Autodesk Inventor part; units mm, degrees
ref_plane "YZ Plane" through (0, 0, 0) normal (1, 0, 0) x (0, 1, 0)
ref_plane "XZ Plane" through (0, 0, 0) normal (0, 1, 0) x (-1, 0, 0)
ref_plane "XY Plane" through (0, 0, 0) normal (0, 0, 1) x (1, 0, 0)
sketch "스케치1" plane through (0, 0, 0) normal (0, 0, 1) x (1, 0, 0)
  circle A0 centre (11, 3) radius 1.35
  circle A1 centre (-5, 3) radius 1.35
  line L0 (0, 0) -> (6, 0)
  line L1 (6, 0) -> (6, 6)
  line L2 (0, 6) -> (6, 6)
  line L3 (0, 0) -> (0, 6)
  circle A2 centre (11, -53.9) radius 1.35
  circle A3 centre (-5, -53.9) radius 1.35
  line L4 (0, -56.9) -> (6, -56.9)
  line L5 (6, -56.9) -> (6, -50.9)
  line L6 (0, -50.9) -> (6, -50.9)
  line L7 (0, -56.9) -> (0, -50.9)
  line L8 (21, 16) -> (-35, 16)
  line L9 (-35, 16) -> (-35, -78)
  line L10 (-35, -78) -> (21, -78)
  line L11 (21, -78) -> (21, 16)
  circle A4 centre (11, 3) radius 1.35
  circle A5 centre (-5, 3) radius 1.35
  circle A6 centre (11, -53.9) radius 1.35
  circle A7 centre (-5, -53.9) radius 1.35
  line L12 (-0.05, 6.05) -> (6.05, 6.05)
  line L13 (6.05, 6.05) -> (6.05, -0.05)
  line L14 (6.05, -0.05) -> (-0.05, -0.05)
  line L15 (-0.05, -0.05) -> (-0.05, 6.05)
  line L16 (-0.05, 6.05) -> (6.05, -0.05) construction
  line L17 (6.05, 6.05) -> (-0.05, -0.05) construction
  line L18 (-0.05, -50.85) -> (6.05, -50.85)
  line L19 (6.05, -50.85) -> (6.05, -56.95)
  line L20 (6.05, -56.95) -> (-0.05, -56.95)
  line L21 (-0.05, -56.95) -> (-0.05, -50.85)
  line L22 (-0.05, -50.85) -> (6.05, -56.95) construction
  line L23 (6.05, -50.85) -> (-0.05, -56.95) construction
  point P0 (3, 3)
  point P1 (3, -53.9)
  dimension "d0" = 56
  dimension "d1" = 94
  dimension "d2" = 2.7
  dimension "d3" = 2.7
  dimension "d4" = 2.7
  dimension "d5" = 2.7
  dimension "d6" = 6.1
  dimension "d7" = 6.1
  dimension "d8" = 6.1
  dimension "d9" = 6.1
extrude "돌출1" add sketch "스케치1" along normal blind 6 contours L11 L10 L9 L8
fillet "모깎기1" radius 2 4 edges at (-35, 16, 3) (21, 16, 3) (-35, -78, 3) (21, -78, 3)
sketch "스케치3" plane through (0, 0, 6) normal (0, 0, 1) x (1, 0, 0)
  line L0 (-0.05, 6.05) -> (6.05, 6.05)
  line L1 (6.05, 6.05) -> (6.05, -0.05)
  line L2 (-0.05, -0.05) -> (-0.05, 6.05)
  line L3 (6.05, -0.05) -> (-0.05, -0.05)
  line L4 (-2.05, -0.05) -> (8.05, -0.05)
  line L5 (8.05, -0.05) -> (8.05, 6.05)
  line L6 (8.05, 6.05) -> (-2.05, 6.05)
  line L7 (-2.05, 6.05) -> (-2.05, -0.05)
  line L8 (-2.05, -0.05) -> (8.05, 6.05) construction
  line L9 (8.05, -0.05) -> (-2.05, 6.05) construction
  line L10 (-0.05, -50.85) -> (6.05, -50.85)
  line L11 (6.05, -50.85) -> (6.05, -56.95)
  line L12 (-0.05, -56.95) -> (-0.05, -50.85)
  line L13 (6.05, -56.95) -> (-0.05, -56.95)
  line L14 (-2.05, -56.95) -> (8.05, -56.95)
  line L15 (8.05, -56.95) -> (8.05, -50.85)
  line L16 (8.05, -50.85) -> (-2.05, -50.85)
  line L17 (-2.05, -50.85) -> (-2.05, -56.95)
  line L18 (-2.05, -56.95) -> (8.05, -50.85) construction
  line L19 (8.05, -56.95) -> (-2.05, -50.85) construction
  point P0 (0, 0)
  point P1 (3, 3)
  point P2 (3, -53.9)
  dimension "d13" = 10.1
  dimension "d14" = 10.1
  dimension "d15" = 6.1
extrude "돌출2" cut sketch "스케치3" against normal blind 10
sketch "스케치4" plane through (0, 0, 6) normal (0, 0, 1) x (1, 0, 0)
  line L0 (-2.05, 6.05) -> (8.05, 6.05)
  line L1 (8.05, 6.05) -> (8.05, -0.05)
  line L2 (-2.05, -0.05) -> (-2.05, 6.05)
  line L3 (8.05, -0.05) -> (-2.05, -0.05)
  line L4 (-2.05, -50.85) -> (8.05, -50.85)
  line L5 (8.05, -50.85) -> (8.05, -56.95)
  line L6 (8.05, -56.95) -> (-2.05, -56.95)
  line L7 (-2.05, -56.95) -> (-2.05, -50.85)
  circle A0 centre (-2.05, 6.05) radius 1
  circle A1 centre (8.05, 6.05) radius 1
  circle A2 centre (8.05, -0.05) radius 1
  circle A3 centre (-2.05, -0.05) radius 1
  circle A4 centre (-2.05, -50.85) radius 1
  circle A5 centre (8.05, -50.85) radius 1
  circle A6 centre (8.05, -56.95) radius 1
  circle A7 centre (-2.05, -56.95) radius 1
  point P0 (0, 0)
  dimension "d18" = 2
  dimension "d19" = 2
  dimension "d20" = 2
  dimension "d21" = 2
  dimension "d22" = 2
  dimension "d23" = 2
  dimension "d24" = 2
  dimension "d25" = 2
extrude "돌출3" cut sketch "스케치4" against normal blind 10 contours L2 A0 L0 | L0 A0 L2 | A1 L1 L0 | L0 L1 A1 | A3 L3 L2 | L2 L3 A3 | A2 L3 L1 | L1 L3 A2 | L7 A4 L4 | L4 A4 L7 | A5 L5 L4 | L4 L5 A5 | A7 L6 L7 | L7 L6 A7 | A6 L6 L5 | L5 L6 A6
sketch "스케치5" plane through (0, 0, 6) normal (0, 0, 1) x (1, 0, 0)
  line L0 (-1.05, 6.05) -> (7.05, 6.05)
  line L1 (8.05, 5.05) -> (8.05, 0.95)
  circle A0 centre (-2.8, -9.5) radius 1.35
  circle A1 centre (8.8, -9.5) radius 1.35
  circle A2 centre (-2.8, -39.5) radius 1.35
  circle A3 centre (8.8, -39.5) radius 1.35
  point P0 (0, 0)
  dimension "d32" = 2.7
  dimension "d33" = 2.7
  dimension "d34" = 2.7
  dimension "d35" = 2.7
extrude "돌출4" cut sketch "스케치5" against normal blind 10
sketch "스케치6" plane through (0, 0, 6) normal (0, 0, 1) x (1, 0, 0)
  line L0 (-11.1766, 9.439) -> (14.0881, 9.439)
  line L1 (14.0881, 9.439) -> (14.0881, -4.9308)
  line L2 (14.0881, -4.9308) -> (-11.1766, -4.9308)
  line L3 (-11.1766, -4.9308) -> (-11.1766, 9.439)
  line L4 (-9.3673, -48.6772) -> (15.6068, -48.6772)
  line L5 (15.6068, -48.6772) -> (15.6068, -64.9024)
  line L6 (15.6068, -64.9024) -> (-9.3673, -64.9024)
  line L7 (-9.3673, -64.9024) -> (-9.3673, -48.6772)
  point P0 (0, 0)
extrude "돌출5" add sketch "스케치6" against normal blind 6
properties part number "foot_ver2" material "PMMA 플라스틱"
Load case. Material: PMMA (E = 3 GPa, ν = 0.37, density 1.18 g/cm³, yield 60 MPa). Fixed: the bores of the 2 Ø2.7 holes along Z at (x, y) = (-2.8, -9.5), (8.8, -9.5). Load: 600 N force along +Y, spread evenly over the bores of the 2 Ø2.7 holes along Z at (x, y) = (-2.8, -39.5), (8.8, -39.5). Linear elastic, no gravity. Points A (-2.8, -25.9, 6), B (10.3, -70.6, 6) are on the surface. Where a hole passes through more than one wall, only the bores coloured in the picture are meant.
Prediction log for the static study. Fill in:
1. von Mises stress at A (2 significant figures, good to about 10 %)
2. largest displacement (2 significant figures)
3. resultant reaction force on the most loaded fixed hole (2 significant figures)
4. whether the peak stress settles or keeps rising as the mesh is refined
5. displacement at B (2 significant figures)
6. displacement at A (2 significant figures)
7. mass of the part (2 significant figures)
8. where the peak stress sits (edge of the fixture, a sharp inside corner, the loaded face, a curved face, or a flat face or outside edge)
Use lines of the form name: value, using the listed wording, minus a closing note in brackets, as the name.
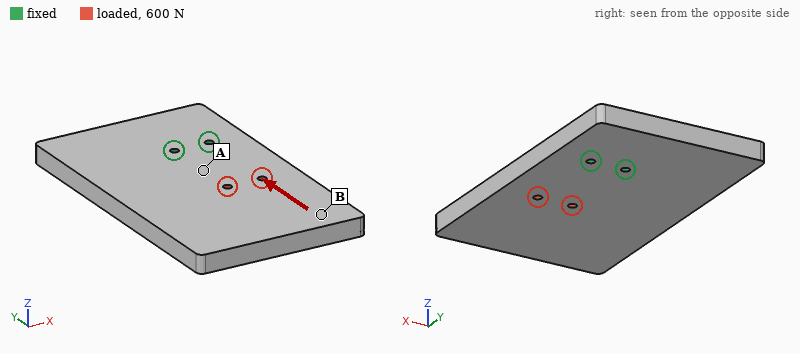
von Mises stress at A: 3.3 MPa
largest displacement: 42 µm
resultant reaction force on the most loaded fixed hole: 300 N
whether the peak stress settles or keeps rising as the mesh is refined: keeps rising
displacement at B: 37 µm
displacement at A: 20 µm
mass of the part: 37 g
where the peak stress sits: edge of the fixture
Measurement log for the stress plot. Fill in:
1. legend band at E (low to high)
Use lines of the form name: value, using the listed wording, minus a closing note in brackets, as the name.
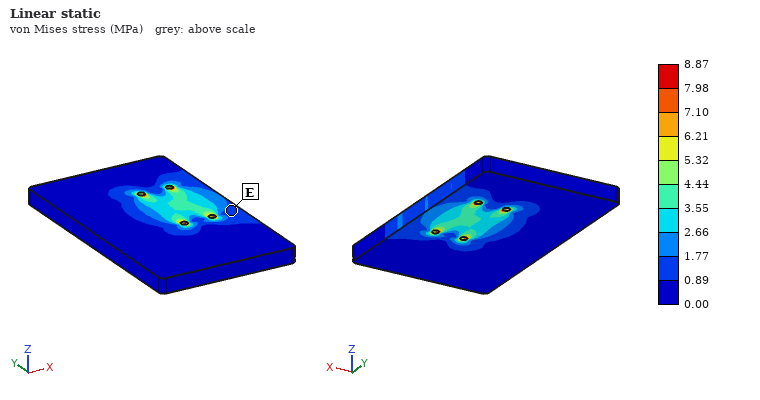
legend band at E: 0.89 to 1.77 MPa
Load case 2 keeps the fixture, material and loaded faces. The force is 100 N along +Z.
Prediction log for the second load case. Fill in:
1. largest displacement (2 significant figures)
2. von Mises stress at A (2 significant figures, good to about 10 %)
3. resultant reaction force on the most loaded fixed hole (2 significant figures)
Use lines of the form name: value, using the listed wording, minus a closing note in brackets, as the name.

largest displacement: 1.3 mm
von Mises stress at A: 4.2 MPa
resultant reaction force on the most loaded fixed hole: 50 N
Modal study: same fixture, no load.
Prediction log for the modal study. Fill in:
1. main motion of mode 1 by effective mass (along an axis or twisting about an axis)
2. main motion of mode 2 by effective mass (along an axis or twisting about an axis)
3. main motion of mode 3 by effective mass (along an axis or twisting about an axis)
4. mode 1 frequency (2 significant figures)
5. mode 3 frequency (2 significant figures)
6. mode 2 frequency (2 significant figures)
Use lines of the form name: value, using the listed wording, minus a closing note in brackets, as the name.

main motion of mode 1 by effective mass: along Z
main motion of mode 2 by effective mass: twisting about Y
main motion of mode 3 by effective mass: along X
mode 1 frequency: 280 Hz
mode 3 frequency: 890 Hz
mode 2 frequency: 710 Hz
